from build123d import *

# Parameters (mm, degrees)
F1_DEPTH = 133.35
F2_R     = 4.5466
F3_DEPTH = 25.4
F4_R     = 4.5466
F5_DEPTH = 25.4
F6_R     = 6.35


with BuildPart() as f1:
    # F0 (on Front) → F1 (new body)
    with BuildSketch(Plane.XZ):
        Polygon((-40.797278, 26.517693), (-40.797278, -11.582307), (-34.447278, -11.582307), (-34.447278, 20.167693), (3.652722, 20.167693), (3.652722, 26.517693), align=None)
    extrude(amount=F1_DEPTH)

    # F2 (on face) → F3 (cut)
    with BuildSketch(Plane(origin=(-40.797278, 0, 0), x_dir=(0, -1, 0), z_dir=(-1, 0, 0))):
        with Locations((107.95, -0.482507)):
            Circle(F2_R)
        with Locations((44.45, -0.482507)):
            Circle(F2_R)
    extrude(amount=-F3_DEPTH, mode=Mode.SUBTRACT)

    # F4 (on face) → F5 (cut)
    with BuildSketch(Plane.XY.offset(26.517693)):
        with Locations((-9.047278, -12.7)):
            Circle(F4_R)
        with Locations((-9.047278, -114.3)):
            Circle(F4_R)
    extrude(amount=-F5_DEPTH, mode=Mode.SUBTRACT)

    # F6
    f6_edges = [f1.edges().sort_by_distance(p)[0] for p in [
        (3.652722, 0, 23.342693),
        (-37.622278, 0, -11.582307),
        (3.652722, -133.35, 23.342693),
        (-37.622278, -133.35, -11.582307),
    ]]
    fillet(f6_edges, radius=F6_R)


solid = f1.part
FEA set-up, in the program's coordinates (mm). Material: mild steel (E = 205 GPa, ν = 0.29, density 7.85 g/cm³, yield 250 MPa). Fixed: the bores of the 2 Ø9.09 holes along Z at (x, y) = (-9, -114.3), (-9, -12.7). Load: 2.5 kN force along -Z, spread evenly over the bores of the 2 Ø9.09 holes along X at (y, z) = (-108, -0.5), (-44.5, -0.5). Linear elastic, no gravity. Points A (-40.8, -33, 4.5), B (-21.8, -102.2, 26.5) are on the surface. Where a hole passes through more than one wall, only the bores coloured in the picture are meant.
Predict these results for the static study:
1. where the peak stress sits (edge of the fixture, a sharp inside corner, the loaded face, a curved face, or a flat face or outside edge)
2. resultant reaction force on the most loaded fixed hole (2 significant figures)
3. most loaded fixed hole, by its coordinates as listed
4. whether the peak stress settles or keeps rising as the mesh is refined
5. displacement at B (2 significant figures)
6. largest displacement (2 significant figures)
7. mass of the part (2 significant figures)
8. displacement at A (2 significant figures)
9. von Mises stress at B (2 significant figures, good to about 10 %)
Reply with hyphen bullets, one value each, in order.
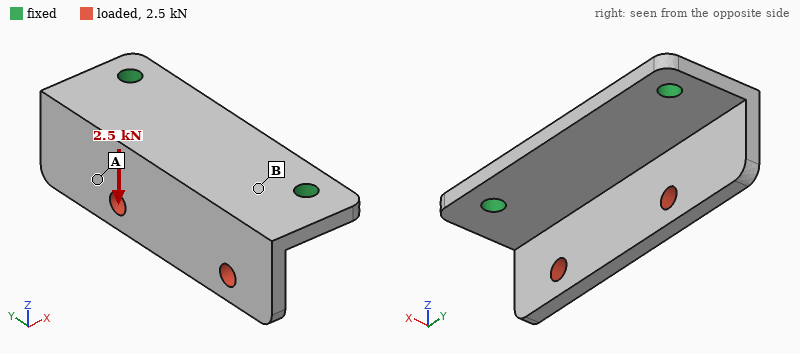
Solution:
- edge of the fixture
- 1.5 kN
- (-9, -114.3)
- keeps rising
- 0.018 mm
- 0.11 mm
- 490 g
- 0.067 mm
- 53 MPa
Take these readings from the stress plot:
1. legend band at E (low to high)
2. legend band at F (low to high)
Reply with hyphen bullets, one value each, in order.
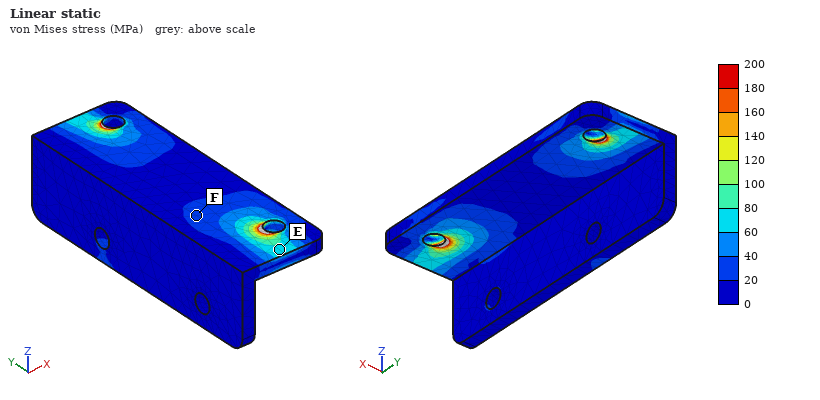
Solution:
- 60 to 80 MPa
- 20 to 40 MPa
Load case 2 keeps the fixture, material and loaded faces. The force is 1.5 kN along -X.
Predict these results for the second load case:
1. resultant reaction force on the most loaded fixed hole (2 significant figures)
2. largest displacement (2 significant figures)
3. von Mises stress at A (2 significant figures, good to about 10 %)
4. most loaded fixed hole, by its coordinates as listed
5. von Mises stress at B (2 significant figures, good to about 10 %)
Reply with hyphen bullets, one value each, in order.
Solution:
- 980 N
- 0.11 mm
- 18 MPa
- (-9, -114.3)
- 41 MPa
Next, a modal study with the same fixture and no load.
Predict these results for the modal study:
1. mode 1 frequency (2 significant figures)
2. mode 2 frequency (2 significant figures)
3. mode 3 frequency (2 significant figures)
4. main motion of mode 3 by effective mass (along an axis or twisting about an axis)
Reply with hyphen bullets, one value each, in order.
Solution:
- 1600 Hz
- 2600 Hz
- 3600 Hz
- along Z
